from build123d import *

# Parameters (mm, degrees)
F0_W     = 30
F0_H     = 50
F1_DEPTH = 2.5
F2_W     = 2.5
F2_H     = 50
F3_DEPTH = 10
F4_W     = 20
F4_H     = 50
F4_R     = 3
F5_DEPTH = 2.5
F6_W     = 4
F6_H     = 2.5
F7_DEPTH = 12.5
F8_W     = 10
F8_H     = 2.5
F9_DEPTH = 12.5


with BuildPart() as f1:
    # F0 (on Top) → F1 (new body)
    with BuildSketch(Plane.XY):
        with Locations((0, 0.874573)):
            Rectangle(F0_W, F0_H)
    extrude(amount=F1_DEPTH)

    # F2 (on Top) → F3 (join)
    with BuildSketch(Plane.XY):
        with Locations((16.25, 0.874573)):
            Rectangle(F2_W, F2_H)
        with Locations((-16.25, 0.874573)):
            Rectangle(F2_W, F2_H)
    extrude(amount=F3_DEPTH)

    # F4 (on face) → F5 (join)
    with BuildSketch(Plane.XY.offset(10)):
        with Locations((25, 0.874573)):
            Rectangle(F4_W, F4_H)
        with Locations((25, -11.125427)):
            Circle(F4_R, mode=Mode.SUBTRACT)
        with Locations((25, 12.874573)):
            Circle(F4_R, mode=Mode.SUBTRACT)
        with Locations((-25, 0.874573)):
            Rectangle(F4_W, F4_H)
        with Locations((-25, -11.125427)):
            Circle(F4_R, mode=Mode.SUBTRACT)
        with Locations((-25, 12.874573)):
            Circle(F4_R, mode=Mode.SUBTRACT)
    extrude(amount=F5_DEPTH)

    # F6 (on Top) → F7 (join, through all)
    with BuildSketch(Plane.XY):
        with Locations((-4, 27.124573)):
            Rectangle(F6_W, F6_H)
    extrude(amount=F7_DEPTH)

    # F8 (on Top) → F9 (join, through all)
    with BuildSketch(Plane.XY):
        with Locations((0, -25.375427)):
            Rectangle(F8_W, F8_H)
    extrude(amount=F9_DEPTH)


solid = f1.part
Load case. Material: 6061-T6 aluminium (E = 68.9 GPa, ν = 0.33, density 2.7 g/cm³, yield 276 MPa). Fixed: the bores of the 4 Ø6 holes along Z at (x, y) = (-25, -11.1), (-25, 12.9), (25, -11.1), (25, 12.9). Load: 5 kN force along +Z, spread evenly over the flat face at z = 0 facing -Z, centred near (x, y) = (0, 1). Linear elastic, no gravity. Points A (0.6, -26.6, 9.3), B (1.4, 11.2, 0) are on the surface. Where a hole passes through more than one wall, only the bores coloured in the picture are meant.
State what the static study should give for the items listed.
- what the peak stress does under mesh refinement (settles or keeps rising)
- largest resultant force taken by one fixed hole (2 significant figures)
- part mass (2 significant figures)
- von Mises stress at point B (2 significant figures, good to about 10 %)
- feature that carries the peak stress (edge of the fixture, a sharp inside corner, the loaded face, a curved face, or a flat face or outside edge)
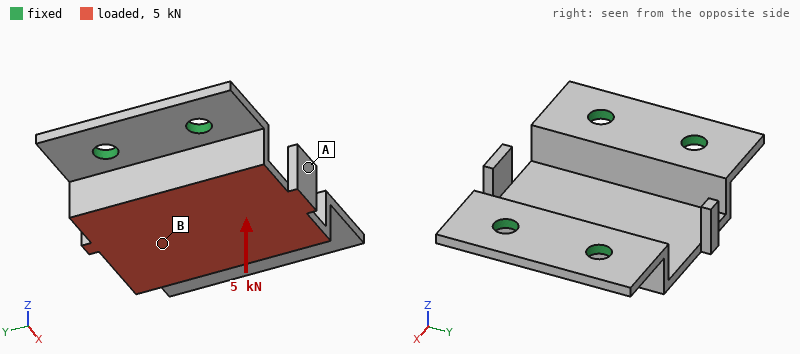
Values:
keeps rising
1.6 kN
31 g
130 MPa
edge of the fixture
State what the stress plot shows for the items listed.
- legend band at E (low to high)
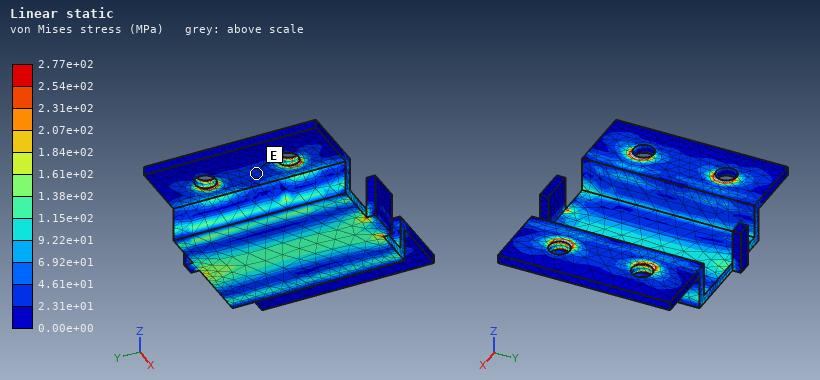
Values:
2.31e+01 to 4.61e+01 MPa
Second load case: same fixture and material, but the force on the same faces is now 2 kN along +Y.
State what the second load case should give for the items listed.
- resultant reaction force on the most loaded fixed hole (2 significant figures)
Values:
760 N
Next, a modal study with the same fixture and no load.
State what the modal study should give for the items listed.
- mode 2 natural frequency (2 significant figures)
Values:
6600 Hz
